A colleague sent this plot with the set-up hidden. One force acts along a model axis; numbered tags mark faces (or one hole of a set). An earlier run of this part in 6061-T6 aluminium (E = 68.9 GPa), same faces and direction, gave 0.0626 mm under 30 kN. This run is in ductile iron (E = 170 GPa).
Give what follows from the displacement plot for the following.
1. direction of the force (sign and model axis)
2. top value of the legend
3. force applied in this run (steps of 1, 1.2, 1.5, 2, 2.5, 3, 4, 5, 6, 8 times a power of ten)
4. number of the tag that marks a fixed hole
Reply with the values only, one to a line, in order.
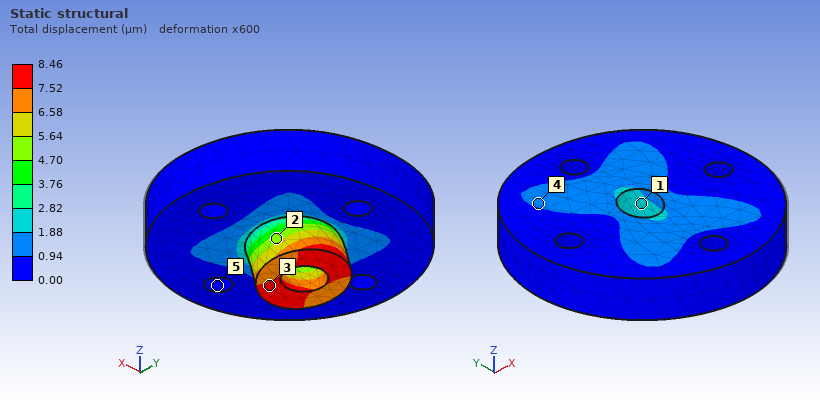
+Y
8.46 µm
10 kN
5
